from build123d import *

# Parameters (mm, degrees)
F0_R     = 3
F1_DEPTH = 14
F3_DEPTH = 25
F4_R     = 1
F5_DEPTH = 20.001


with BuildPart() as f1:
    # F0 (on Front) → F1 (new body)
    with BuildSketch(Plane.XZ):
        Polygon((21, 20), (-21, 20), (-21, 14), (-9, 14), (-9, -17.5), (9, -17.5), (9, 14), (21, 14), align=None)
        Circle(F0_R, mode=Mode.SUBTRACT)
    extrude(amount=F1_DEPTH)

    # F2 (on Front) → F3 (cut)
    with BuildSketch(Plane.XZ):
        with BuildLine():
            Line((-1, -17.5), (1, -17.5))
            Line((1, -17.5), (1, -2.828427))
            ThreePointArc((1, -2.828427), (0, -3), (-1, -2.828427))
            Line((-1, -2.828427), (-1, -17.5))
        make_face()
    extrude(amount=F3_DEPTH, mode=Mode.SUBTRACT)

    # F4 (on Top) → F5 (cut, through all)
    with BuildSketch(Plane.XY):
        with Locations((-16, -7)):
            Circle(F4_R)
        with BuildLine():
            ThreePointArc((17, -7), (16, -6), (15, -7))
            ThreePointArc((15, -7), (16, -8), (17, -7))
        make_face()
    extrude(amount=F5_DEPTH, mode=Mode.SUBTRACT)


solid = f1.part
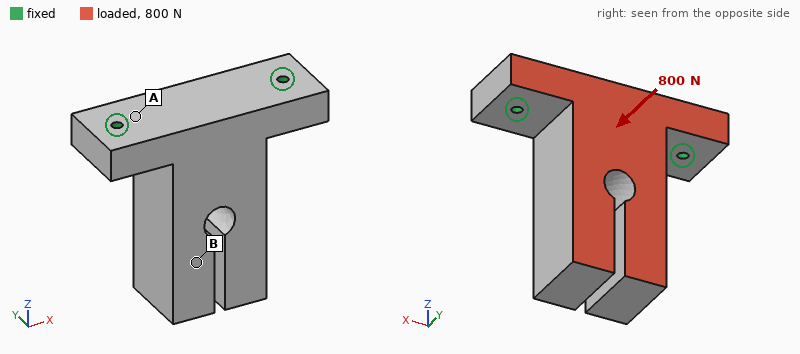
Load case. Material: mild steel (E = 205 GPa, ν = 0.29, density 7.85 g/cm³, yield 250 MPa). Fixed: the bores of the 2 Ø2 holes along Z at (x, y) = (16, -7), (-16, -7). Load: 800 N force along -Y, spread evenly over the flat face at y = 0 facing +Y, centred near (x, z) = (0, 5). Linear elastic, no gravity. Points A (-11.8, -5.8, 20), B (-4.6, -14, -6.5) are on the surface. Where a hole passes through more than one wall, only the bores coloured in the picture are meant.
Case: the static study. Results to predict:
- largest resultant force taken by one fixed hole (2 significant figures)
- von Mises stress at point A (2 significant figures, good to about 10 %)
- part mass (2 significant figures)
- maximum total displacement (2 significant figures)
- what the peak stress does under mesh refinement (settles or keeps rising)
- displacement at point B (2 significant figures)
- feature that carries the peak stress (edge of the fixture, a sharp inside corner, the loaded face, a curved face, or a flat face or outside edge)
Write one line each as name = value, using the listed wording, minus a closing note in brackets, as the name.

largest resultant force taken by one fixed hole = 400 N
von Mises stress at point A = 37 MPa
part mass = 83 g
maximum total displacement = 35 µm
what the peak stress does under mesh refinement = keeps rising
displacement at point B = 24 µm
feature that carries the peak stress = edge of the fixture
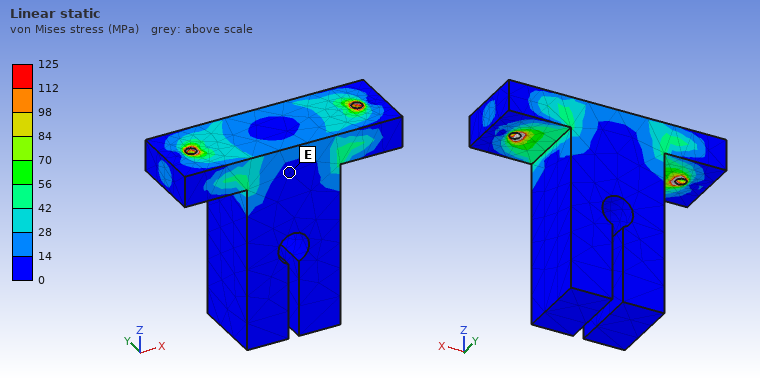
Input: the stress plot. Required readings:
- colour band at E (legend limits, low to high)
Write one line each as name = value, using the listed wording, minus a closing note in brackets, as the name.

colour band at E = 0 to 14 MPa
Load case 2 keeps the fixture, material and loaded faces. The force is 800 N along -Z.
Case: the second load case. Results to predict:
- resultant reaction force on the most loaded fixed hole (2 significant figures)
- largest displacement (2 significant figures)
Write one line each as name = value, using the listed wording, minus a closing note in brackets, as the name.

resultant reaction force on the most loaded fixed hole = 410 N
largest displacement = 17 µm
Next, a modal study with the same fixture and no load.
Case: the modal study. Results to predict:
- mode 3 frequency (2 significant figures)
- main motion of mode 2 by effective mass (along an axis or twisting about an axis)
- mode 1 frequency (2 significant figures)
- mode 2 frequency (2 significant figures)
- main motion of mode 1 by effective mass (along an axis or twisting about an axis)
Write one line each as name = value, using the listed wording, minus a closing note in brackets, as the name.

mode 3 frequency = 8300 Hz
main motion of mode 2 by effective mass = along X
mode 1 frequency = 3200 Hz
mode 2 frequency = 6100 Hz
main motion of mode 1 by effective mass = along Y
